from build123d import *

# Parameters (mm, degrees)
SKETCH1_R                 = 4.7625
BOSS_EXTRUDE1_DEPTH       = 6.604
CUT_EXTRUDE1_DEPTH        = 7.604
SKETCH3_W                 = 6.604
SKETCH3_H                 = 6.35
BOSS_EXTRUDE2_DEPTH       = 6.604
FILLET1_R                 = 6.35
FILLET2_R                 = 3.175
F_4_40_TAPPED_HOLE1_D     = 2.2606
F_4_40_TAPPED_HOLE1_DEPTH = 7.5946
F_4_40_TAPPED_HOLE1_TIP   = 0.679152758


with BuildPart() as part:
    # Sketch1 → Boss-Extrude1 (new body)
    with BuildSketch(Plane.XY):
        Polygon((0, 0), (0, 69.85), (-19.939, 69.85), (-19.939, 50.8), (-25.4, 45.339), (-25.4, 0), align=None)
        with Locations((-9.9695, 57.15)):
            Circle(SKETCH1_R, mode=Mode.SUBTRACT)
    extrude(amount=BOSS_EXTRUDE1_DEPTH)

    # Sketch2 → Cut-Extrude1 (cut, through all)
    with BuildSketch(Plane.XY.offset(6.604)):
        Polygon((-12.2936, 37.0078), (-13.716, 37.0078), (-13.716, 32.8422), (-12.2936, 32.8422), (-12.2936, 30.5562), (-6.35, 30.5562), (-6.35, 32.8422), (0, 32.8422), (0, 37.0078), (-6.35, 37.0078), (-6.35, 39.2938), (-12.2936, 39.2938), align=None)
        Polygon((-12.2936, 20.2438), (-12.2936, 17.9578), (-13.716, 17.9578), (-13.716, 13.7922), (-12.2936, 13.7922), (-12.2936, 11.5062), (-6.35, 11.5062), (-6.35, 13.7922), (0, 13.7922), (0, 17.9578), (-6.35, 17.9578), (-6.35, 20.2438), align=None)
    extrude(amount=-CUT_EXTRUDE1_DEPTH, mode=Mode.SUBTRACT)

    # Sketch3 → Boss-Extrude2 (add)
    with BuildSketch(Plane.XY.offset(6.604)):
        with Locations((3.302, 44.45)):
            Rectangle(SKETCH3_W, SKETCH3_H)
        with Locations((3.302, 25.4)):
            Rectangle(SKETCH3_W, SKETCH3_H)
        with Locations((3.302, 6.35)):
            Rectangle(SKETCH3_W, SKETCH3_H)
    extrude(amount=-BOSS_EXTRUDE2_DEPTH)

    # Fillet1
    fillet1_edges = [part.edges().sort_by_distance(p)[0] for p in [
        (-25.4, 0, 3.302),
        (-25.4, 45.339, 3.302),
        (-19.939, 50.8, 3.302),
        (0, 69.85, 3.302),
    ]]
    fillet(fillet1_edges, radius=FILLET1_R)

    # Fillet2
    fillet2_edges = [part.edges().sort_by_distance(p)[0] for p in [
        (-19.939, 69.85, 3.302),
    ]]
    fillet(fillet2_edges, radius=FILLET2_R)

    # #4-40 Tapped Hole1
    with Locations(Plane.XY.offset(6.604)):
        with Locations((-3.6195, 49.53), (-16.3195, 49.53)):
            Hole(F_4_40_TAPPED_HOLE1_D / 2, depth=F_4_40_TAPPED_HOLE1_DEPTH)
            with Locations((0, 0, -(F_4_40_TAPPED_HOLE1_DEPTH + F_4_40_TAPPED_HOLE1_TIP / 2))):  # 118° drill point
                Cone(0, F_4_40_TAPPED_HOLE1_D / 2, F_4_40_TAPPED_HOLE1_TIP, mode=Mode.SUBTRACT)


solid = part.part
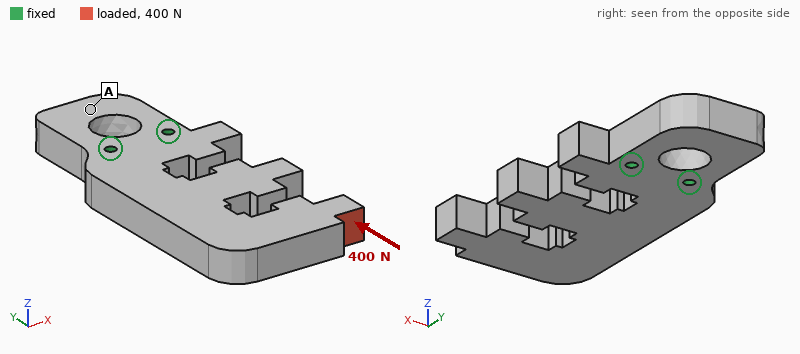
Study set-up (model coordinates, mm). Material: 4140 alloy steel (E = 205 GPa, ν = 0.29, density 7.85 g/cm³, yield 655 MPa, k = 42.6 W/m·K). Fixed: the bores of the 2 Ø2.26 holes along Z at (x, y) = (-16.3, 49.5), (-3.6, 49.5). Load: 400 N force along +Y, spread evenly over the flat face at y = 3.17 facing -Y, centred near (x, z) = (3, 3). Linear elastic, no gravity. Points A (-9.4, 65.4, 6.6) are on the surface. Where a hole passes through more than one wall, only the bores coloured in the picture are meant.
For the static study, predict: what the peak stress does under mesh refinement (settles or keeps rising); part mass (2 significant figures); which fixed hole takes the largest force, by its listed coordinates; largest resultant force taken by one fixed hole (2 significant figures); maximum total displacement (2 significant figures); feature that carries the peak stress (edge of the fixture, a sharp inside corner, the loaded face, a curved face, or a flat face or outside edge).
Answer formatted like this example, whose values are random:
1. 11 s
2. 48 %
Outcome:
1. keeps rising
2. 78 g
3. (-3.6, 49.5)
4. 660 N
5. 66 µm
6. a sharp inside corner
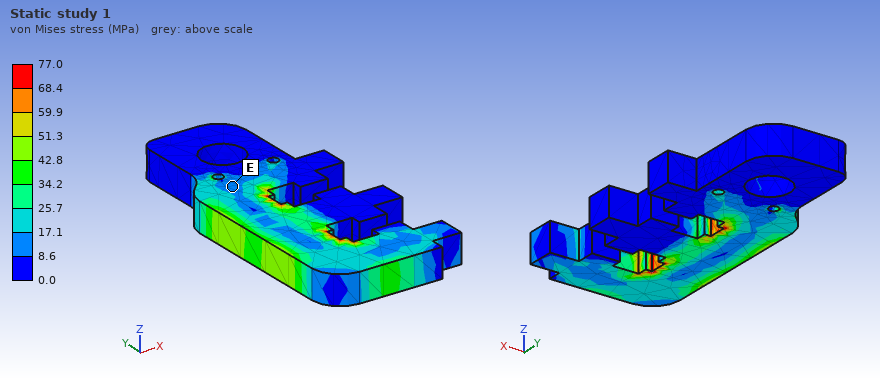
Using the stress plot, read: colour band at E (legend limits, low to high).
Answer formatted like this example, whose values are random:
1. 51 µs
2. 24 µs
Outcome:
1. 8.6 to 17.1 MPa
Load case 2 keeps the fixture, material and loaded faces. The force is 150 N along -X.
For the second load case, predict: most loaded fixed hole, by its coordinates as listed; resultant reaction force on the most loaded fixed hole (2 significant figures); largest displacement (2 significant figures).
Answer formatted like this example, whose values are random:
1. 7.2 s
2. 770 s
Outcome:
1. (-3.6, 49.5)
2. 570 N
3. 29 µm
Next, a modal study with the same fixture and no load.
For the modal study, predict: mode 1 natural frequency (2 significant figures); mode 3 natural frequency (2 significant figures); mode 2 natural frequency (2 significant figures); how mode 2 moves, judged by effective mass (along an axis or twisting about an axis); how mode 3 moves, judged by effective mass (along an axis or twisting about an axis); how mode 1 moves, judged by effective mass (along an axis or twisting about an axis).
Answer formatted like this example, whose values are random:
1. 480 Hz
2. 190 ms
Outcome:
1. 1500 Hz
2. 4300 Hz
3. 2700 Hz
4. along X
5. twisting about Y
6. along Z
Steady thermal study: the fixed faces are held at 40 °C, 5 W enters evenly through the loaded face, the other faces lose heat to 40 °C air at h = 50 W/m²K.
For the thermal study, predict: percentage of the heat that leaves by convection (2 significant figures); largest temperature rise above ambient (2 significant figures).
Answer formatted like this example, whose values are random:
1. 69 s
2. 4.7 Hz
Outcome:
1. 64 %
2. 60 K
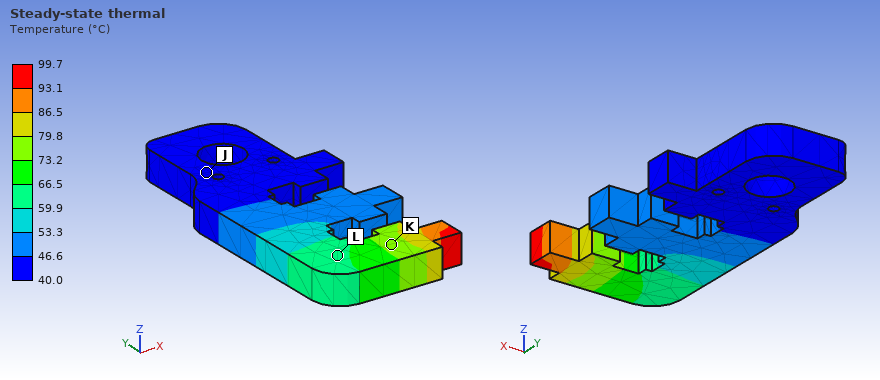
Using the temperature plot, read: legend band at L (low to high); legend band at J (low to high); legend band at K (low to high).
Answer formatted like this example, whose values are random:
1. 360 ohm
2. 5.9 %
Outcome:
1. 59.9 to 66.5 °C
2. 40.0 to 46.6 °C
3. 73.2 to 79.8 °C
